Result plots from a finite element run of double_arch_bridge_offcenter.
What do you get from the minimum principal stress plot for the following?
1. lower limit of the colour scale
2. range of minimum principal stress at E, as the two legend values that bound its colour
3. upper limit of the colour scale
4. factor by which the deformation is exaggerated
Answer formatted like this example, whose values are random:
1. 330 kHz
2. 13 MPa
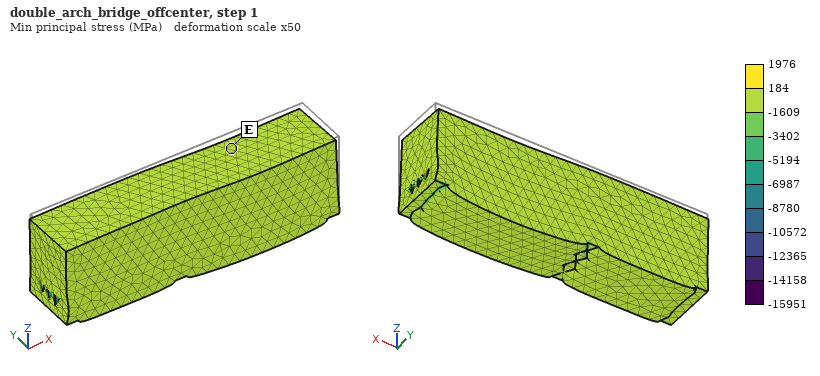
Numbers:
1. -15951 MPa
2. -1609 to 184 MPa
3. 1976 MPa
4. 50
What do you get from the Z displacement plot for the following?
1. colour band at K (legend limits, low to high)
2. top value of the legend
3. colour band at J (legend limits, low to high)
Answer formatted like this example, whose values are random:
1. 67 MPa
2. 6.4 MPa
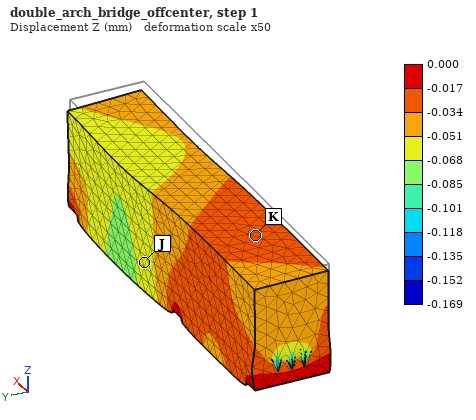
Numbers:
1. -0.034 to -0.017 mm
2. 0.000 mm
3. -0.068 to -0.051 mm
